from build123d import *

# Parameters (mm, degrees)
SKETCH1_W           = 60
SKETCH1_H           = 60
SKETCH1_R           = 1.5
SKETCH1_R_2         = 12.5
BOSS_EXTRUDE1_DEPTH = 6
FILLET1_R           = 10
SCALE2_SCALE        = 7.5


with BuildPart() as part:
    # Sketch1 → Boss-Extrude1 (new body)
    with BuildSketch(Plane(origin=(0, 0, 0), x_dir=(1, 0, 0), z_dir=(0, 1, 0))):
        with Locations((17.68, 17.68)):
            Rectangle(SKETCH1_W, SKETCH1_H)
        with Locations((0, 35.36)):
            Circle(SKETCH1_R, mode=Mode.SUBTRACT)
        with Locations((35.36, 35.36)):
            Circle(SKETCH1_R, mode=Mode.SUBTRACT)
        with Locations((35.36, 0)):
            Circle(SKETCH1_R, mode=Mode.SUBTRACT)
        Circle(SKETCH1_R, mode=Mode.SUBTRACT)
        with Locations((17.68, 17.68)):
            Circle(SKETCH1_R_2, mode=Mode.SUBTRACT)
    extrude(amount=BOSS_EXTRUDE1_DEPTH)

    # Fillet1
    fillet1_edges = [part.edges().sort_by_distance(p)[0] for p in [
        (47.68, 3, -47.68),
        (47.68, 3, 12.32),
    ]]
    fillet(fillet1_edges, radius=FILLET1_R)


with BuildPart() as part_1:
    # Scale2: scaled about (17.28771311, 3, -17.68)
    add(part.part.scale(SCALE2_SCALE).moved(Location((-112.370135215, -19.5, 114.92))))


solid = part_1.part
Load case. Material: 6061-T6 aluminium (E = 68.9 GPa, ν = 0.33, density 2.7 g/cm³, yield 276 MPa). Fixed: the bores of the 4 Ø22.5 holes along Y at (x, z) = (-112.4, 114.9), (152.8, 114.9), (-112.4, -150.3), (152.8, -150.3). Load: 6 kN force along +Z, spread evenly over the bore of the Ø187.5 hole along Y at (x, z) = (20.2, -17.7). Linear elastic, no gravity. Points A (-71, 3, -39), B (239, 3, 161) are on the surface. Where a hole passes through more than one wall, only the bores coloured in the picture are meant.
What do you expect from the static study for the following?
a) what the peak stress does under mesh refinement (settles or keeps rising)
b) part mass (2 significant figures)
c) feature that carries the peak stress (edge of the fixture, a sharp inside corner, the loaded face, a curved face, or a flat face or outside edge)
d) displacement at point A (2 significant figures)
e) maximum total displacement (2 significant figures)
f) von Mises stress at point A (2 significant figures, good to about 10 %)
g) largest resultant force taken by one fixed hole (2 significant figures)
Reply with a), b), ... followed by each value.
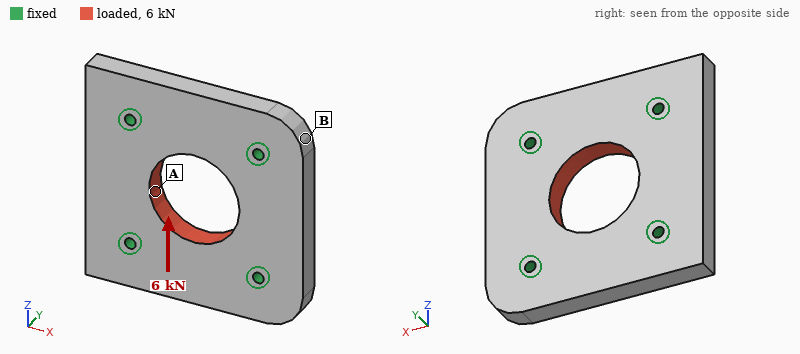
a) keeps rising
b) 21 kg
c) edge of the fixture
d) 0.54 µm
e) 0.91 µm
f) 0.40 MPa
g) 1.5 kN
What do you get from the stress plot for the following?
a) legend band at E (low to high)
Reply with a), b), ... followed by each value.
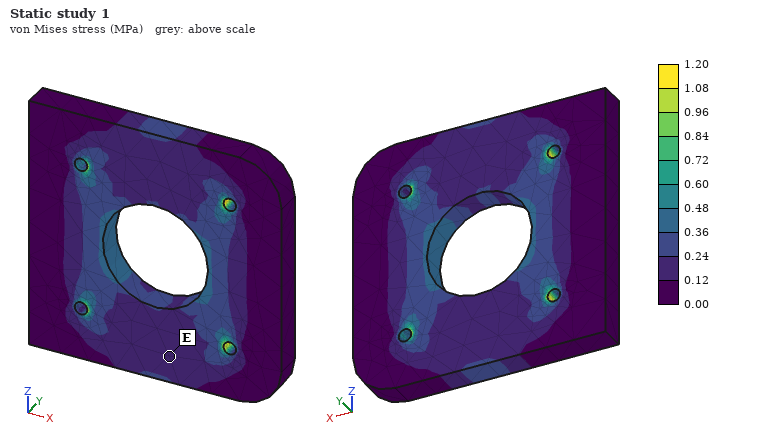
a) 0.12 to 0.24 MPa
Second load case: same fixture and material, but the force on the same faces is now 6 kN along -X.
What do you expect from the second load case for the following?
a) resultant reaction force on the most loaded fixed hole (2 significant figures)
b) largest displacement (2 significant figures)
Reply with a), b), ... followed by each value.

a) 1.5 kN
b) 0.91 µm
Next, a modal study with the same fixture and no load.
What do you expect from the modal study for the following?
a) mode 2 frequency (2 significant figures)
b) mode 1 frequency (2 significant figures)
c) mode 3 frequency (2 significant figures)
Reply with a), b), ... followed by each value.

a) 2200 Hz
b) 1900 Hz
c) 2200 Hz
